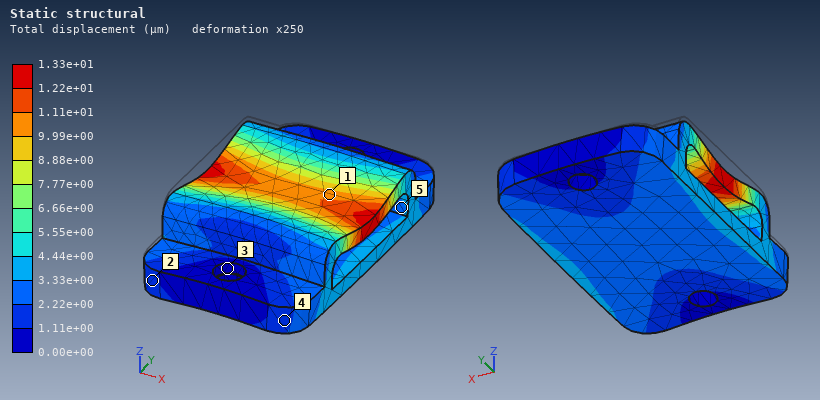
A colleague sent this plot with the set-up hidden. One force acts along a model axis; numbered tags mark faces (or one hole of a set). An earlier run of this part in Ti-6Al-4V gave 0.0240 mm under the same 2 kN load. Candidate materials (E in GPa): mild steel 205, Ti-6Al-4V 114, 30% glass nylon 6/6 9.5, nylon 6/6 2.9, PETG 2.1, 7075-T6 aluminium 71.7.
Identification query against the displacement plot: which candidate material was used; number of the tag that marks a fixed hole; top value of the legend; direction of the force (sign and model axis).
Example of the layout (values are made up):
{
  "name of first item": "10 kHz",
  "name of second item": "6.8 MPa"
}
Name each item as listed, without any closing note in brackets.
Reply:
{
  "which candidate material was used": "mild steel",
  "number of the tag that marks a fixed hole": "3",
  "top value of the legend": "1.33e+01 µm",
  "direction of the force": "-Z"
}
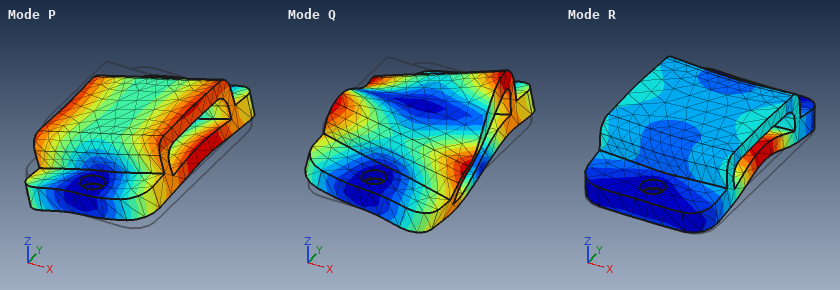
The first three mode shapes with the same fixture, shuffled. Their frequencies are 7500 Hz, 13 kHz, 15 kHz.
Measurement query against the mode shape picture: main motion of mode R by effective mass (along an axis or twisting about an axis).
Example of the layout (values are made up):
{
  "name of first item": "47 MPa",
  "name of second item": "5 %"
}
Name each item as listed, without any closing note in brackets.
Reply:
{
  "main motion of mode R by effective mass": "along Z"
}
